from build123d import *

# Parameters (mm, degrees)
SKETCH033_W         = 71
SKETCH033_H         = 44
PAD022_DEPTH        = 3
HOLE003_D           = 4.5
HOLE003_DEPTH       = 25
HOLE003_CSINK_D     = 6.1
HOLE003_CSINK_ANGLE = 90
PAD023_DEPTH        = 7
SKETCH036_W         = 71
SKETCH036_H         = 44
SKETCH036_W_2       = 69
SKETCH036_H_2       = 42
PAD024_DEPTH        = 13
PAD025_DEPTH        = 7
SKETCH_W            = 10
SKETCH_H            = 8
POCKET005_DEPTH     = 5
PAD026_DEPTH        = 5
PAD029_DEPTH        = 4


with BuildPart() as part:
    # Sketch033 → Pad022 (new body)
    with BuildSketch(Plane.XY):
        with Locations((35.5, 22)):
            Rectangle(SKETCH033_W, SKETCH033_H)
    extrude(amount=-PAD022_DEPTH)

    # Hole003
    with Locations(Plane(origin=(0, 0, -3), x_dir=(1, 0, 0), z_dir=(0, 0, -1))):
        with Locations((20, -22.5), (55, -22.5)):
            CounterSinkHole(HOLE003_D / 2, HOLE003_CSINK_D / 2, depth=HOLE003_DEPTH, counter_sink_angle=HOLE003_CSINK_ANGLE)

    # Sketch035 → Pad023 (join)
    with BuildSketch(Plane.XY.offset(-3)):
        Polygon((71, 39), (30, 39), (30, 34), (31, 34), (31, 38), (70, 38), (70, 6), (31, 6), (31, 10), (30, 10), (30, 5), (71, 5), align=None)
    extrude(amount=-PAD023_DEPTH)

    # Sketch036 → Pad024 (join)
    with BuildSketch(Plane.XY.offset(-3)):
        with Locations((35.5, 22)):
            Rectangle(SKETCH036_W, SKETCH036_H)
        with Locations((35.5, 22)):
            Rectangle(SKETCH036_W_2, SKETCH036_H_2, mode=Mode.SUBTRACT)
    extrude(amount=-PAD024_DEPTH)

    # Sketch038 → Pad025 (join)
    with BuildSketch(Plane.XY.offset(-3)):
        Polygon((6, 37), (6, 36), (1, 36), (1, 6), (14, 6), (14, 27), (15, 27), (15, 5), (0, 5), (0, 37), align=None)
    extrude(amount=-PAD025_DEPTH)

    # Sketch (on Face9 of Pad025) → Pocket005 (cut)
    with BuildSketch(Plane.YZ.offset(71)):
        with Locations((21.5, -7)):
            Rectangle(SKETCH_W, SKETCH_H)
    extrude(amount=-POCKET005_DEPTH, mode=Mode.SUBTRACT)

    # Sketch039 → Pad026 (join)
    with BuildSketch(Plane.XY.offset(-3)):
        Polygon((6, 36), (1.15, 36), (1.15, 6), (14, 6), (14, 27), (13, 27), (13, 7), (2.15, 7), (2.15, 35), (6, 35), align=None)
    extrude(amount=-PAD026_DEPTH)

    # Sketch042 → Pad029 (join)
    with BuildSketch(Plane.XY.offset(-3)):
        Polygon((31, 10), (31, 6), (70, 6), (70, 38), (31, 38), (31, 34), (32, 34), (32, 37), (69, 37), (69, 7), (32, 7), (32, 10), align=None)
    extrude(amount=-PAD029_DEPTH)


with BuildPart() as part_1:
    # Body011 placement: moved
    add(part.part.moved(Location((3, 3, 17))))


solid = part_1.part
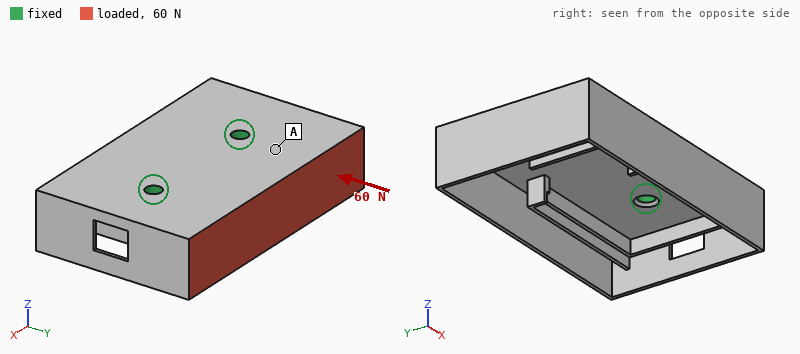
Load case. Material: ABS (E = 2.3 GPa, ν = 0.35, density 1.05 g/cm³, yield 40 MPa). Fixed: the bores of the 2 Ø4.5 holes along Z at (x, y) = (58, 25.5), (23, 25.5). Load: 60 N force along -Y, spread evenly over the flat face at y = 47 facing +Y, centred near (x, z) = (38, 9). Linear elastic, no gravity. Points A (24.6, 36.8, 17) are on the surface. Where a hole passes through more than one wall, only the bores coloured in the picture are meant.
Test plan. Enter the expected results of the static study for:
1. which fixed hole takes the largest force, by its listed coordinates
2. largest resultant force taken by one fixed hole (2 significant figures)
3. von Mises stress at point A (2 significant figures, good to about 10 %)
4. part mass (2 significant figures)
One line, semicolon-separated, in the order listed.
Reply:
(23, 25.5); 34 N; 2.0 MPa; 14 g
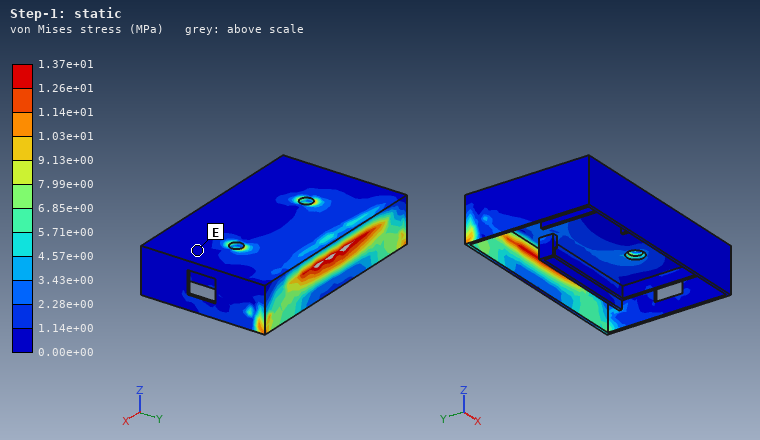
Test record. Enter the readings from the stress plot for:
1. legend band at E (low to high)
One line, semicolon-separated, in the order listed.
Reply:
0.00e+00 to 1.14e+00 MPa
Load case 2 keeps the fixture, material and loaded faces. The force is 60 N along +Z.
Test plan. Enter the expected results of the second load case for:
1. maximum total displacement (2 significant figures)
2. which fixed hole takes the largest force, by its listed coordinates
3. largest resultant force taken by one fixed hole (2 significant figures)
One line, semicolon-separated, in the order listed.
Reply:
0.80 mm; (23, 25.5); 33 N
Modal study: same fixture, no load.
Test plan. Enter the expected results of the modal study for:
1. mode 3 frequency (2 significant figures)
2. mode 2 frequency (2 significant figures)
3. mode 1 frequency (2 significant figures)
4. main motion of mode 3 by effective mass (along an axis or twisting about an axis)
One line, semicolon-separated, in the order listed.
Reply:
1200 Hz; 870 Hz; 740 Hz; along Z
